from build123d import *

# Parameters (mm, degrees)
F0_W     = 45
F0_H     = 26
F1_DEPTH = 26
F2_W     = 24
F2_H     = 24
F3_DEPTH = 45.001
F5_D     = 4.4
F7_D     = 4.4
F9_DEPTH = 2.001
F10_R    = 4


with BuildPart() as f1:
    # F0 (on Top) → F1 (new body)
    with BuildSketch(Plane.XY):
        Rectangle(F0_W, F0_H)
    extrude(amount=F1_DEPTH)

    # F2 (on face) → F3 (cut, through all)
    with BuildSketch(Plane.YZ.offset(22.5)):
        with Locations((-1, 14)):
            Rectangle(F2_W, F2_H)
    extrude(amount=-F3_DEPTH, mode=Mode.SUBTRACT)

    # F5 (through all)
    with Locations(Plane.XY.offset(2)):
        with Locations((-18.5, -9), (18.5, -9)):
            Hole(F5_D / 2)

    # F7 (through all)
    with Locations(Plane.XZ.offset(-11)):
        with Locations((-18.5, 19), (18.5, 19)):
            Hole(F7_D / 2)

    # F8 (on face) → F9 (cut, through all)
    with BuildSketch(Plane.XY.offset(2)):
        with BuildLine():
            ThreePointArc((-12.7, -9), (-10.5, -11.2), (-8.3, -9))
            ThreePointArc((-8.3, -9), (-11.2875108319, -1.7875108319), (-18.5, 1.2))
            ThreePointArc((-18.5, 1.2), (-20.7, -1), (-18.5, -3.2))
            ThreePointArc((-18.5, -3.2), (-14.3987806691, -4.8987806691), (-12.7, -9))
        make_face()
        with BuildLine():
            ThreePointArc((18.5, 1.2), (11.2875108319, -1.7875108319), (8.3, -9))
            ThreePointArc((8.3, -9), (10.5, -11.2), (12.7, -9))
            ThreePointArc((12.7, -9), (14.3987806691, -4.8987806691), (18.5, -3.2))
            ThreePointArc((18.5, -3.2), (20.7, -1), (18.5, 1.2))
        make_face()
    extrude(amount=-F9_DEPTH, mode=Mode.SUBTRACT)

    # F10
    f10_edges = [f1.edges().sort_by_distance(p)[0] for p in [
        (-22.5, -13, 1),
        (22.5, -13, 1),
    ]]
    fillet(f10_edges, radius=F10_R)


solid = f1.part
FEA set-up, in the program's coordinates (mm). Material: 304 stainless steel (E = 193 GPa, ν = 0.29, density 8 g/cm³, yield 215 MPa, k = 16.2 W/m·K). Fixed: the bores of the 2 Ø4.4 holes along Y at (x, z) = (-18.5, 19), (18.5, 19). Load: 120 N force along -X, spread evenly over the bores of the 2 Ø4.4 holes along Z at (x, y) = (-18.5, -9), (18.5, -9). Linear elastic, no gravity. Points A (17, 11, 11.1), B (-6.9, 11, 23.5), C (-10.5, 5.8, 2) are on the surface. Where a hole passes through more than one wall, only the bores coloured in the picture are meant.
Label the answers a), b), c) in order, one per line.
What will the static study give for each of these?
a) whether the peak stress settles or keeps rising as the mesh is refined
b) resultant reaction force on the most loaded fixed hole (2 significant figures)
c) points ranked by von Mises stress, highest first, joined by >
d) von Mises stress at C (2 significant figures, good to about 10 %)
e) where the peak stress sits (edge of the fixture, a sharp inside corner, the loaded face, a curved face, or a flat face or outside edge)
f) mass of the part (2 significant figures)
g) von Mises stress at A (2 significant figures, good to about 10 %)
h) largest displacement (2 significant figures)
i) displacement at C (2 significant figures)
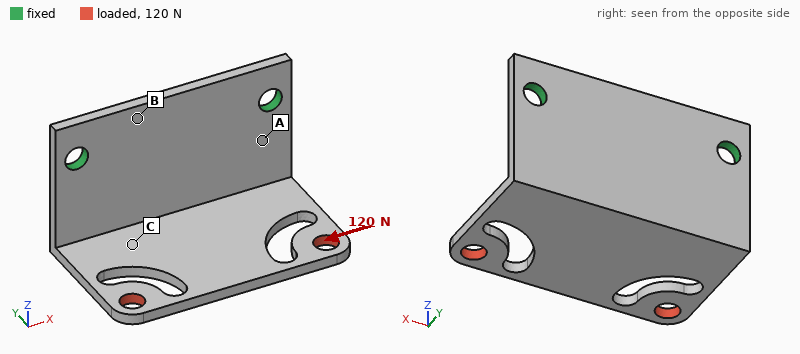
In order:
a) keeps rising
b) 110 N
c) A > C > B
d) 22 MPa
e) edge of the fixture
f) 33 g
g) 36 MPa
h) 53 µm
i) 18 µm
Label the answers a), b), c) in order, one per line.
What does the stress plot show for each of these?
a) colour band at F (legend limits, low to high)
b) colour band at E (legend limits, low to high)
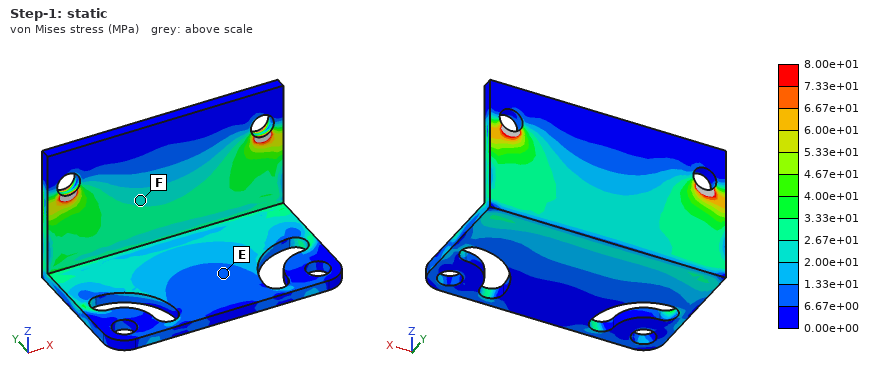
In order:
a) 2.00e+01 to 2.67e+01 MPa
b) 6.67e+00 to 1.33e+01 MPa
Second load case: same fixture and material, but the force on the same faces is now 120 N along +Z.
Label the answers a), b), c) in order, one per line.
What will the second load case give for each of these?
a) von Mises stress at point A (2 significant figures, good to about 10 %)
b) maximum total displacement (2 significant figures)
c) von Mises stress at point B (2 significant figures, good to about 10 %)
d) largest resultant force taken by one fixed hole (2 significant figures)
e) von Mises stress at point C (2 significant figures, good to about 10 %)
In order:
a) 90 MPa
b) 0.32 mm
c) 27 MPa
d) 62 N
e) 50 MPa
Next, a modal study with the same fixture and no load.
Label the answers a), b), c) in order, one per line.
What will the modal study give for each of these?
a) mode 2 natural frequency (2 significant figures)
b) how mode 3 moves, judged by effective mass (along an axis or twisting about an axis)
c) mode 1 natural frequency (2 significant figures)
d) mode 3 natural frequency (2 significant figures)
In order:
a) 2600 Hz
b) along Y
c) 1200 Hz
d) 3300 Hz
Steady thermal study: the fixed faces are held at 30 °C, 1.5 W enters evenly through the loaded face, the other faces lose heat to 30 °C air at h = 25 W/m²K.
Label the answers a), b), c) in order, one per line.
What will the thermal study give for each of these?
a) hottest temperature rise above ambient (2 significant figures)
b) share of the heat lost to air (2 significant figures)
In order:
a) 50 K
b) 75 %
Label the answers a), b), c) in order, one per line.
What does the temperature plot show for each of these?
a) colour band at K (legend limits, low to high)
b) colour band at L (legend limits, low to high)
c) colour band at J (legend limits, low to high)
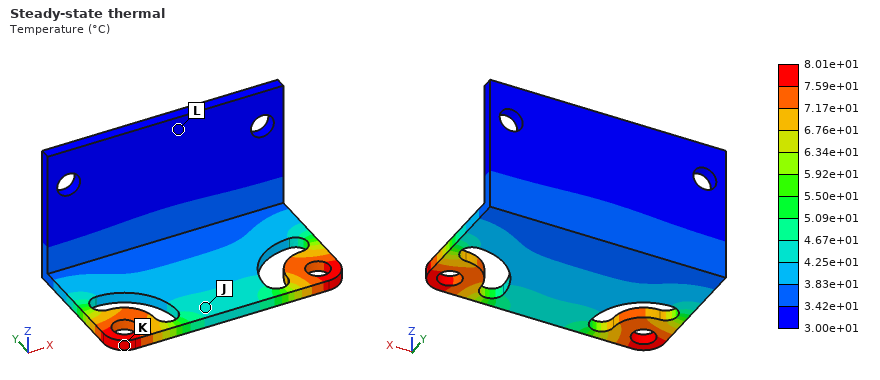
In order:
a) 7.59e+01 to 8.01e+01 °C
b) 3.00e+01 to 3.42e+01 °C
c) 4.25e+01 to 4.67e+01 °C
